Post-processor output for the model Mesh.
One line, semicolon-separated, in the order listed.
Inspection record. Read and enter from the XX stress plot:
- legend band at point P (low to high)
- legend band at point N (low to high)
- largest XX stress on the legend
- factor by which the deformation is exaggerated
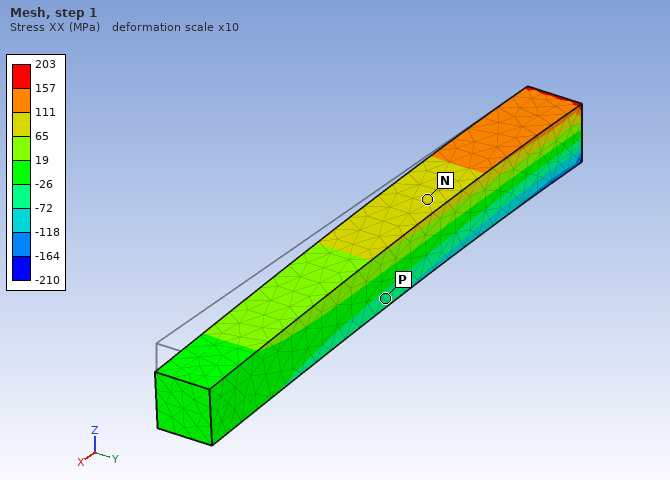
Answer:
-72 to -26 MPa; 65 to 111 MPa; 203 MPa; 10
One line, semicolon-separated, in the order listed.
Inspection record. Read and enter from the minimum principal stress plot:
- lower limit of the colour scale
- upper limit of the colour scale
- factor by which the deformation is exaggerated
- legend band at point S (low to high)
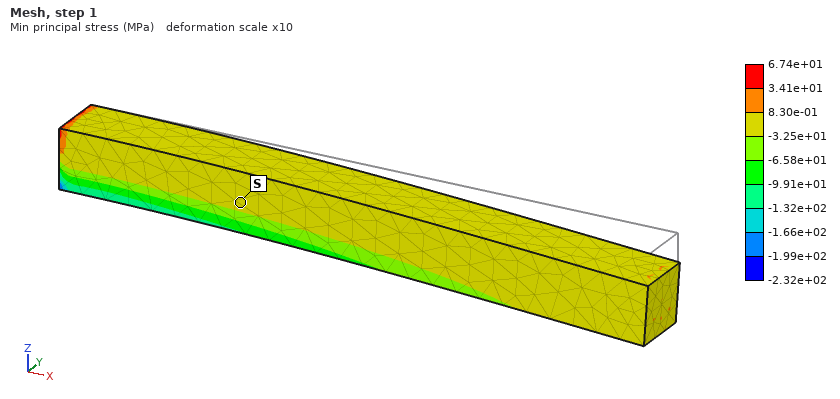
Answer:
-2.32e+02 MPa; 6.74e+01 MPa; 10; -3.25e+01 to 8.30e-01 MPa
